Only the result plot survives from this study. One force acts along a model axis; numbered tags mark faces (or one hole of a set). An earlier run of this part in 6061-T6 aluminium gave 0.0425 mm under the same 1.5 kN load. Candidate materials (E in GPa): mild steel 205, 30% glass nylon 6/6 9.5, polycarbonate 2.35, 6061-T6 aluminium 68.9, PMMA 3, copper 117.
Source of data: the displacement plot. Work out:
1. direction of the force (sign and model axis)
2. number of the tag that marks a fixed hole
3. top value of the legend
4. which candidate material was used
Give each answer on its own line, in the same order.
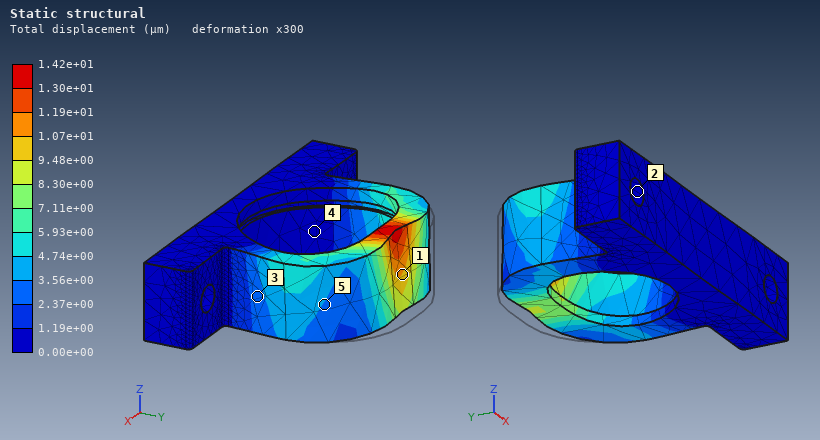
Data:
-Y
2
1.42e+01 µm
mild steel
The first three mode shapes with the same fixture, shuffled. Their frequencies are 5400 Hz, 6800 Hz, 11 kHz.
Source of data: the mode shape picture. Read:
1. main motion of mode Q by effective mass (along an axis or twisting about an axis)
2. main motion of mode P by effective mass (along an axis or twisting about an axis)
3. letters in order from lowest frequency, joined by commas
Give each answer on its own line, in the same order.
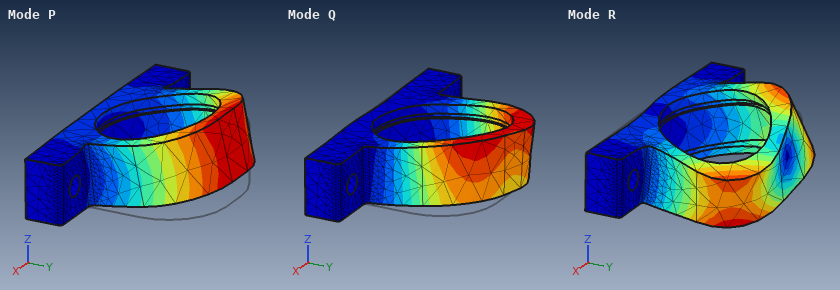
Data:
along X
along Z
P, Q, R
